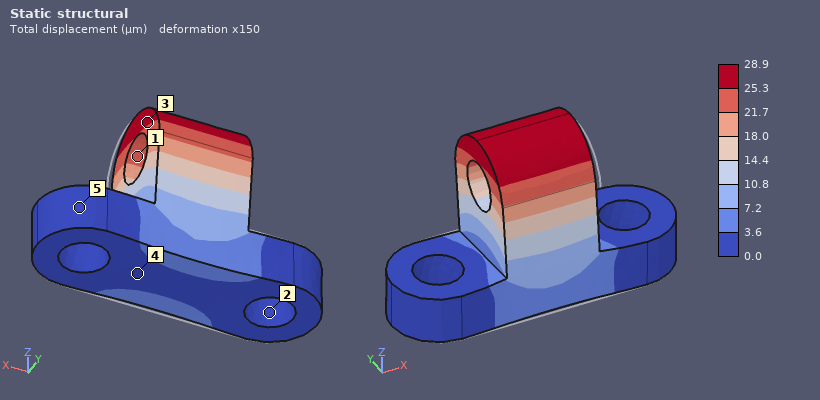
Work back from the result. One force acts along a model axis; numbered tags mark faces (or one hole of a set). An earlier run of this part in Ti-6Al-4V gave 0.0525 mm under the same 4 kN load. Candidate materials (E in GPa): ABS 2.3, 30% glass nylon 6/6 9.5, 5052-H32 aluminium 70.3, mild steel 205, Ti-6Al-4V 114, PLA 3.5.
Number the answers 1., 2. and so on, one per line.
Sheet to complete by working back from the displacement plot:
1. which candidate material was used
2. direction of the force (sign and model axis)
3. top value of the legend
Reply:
1. mild steel
2. +Y
3. 28.9 µm
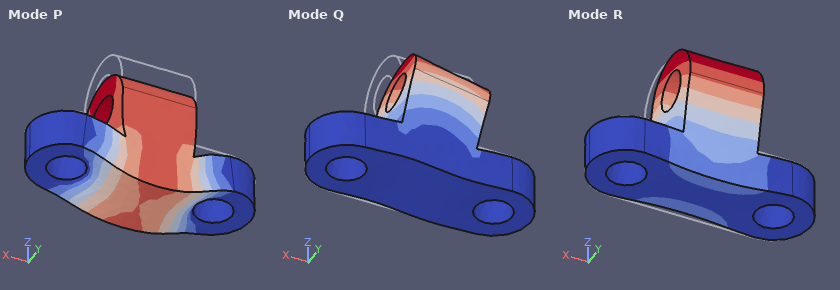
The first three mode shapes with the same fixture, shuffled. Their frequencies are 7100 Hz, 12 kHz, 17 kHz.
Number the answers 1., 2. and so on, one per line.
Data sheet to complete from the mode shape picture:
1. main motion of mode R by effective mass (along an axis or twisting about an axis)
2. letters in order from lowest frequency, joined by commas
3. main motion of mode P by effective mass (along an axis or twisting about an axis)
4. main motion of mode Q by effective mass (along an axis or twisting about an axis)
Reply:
1. along Y
2. R, Q, P
3. along Z
4. along X
